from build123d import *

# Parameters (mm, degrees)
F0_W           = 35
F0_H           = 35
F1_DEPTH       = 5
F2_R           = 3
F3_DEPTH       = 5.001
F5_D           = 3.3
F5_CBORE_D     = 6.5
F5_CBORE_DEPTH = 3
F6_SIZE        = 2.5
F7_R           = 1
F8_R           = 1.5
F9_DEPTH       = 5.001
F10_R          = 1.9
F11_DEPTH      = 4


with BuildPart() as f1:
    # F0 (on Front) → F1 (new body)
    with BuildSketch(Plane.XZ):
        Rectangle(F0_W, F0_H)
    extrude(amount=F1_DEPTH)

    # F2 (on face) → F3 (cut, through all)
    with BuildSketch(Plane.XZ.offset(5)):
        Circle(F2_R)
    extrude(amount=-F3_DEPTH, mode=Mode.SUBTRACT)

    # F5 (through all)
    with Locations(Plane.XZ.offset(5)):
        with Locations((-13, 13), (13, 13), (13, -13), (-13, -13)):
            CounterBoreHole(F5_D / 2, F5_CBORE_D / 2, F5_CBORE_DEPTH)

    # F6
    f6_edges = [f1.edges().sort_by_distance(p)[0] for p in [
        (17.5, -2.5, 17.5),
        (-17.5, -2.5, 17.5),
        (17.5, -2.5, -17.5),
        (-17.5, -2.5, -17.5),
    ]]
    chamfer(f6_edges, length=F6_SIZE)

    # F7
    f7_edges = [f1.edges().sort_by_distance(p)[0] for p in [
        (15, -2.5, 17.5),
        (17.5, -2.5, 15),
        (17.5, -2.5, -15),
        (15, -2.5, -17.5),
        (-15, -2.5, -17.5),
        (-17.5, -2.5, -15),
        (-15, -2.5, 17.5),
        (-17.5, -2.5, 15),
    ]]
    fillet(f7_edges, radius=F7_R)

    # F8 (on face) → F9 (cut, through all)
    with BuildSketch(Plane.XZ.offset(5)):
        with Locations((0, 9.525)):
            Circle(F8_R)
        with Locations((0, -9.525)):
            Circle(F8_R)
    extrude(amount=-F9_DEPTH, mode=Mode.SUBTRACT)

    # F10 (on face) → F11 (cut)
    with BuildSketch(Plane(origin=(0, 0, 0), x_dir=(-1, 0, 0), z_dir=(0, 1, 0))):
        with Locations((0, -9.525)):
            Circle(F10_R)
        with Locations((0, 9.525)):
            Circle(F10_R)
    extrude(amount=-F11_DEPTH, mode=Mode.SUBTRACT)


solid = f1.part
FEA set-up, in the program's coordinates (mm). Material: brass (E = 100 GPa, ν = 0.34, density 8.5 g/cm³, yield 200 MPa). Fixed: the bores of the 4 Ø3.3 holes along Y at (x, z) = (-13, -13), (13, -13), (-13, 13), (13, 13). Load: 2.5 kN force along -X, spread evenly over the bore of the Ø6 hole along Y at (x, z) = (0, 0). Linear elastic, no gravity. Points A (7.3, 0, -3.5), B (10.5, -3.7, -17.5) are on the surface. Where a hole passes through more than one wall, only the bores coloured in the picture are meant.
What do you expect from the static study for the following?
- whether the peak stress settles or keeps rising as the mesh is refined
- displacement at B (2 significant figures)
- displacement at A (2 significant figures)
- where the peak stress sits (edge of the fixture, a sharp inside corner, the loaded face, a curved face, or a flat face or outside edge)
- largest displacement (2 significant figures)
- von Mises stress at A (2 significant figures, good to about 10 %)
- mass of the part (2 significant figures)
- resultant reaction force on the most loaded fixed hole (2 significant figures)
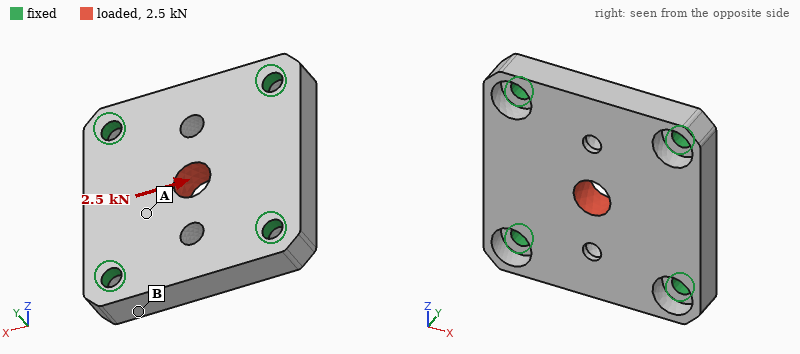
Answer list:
keeps rising
0.98 µm
3.5 µm
edge of the fixture
4.8 µm
18 MPa
45 g
670 N
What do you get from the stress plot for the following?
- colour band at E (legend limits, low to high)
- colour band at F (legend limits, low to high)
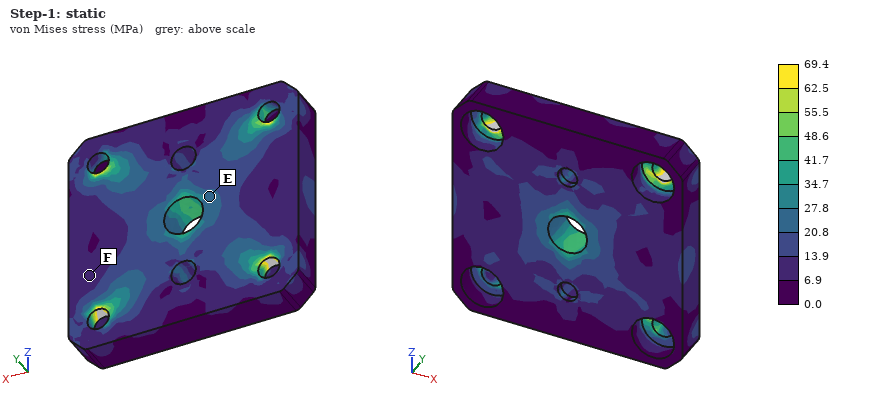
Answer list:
20.8 to 27.8 MPa
6.9 to 13.9 MPa
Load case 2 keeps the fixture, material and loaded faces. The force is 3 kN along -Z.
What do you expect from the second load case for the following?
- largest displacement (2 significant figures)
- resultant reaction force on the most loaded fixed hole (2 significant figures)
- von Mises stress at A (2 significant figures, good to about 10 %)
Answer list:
5.9 µm
810 N
20 MPa
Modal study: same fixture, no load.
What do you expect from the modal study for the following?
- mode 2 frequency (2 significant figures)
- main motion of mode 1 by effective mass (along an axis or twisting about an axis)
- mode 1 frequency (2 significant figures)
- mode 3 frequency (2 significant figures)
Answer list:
18 kHz
along Y
13 kHz
18 kHz
